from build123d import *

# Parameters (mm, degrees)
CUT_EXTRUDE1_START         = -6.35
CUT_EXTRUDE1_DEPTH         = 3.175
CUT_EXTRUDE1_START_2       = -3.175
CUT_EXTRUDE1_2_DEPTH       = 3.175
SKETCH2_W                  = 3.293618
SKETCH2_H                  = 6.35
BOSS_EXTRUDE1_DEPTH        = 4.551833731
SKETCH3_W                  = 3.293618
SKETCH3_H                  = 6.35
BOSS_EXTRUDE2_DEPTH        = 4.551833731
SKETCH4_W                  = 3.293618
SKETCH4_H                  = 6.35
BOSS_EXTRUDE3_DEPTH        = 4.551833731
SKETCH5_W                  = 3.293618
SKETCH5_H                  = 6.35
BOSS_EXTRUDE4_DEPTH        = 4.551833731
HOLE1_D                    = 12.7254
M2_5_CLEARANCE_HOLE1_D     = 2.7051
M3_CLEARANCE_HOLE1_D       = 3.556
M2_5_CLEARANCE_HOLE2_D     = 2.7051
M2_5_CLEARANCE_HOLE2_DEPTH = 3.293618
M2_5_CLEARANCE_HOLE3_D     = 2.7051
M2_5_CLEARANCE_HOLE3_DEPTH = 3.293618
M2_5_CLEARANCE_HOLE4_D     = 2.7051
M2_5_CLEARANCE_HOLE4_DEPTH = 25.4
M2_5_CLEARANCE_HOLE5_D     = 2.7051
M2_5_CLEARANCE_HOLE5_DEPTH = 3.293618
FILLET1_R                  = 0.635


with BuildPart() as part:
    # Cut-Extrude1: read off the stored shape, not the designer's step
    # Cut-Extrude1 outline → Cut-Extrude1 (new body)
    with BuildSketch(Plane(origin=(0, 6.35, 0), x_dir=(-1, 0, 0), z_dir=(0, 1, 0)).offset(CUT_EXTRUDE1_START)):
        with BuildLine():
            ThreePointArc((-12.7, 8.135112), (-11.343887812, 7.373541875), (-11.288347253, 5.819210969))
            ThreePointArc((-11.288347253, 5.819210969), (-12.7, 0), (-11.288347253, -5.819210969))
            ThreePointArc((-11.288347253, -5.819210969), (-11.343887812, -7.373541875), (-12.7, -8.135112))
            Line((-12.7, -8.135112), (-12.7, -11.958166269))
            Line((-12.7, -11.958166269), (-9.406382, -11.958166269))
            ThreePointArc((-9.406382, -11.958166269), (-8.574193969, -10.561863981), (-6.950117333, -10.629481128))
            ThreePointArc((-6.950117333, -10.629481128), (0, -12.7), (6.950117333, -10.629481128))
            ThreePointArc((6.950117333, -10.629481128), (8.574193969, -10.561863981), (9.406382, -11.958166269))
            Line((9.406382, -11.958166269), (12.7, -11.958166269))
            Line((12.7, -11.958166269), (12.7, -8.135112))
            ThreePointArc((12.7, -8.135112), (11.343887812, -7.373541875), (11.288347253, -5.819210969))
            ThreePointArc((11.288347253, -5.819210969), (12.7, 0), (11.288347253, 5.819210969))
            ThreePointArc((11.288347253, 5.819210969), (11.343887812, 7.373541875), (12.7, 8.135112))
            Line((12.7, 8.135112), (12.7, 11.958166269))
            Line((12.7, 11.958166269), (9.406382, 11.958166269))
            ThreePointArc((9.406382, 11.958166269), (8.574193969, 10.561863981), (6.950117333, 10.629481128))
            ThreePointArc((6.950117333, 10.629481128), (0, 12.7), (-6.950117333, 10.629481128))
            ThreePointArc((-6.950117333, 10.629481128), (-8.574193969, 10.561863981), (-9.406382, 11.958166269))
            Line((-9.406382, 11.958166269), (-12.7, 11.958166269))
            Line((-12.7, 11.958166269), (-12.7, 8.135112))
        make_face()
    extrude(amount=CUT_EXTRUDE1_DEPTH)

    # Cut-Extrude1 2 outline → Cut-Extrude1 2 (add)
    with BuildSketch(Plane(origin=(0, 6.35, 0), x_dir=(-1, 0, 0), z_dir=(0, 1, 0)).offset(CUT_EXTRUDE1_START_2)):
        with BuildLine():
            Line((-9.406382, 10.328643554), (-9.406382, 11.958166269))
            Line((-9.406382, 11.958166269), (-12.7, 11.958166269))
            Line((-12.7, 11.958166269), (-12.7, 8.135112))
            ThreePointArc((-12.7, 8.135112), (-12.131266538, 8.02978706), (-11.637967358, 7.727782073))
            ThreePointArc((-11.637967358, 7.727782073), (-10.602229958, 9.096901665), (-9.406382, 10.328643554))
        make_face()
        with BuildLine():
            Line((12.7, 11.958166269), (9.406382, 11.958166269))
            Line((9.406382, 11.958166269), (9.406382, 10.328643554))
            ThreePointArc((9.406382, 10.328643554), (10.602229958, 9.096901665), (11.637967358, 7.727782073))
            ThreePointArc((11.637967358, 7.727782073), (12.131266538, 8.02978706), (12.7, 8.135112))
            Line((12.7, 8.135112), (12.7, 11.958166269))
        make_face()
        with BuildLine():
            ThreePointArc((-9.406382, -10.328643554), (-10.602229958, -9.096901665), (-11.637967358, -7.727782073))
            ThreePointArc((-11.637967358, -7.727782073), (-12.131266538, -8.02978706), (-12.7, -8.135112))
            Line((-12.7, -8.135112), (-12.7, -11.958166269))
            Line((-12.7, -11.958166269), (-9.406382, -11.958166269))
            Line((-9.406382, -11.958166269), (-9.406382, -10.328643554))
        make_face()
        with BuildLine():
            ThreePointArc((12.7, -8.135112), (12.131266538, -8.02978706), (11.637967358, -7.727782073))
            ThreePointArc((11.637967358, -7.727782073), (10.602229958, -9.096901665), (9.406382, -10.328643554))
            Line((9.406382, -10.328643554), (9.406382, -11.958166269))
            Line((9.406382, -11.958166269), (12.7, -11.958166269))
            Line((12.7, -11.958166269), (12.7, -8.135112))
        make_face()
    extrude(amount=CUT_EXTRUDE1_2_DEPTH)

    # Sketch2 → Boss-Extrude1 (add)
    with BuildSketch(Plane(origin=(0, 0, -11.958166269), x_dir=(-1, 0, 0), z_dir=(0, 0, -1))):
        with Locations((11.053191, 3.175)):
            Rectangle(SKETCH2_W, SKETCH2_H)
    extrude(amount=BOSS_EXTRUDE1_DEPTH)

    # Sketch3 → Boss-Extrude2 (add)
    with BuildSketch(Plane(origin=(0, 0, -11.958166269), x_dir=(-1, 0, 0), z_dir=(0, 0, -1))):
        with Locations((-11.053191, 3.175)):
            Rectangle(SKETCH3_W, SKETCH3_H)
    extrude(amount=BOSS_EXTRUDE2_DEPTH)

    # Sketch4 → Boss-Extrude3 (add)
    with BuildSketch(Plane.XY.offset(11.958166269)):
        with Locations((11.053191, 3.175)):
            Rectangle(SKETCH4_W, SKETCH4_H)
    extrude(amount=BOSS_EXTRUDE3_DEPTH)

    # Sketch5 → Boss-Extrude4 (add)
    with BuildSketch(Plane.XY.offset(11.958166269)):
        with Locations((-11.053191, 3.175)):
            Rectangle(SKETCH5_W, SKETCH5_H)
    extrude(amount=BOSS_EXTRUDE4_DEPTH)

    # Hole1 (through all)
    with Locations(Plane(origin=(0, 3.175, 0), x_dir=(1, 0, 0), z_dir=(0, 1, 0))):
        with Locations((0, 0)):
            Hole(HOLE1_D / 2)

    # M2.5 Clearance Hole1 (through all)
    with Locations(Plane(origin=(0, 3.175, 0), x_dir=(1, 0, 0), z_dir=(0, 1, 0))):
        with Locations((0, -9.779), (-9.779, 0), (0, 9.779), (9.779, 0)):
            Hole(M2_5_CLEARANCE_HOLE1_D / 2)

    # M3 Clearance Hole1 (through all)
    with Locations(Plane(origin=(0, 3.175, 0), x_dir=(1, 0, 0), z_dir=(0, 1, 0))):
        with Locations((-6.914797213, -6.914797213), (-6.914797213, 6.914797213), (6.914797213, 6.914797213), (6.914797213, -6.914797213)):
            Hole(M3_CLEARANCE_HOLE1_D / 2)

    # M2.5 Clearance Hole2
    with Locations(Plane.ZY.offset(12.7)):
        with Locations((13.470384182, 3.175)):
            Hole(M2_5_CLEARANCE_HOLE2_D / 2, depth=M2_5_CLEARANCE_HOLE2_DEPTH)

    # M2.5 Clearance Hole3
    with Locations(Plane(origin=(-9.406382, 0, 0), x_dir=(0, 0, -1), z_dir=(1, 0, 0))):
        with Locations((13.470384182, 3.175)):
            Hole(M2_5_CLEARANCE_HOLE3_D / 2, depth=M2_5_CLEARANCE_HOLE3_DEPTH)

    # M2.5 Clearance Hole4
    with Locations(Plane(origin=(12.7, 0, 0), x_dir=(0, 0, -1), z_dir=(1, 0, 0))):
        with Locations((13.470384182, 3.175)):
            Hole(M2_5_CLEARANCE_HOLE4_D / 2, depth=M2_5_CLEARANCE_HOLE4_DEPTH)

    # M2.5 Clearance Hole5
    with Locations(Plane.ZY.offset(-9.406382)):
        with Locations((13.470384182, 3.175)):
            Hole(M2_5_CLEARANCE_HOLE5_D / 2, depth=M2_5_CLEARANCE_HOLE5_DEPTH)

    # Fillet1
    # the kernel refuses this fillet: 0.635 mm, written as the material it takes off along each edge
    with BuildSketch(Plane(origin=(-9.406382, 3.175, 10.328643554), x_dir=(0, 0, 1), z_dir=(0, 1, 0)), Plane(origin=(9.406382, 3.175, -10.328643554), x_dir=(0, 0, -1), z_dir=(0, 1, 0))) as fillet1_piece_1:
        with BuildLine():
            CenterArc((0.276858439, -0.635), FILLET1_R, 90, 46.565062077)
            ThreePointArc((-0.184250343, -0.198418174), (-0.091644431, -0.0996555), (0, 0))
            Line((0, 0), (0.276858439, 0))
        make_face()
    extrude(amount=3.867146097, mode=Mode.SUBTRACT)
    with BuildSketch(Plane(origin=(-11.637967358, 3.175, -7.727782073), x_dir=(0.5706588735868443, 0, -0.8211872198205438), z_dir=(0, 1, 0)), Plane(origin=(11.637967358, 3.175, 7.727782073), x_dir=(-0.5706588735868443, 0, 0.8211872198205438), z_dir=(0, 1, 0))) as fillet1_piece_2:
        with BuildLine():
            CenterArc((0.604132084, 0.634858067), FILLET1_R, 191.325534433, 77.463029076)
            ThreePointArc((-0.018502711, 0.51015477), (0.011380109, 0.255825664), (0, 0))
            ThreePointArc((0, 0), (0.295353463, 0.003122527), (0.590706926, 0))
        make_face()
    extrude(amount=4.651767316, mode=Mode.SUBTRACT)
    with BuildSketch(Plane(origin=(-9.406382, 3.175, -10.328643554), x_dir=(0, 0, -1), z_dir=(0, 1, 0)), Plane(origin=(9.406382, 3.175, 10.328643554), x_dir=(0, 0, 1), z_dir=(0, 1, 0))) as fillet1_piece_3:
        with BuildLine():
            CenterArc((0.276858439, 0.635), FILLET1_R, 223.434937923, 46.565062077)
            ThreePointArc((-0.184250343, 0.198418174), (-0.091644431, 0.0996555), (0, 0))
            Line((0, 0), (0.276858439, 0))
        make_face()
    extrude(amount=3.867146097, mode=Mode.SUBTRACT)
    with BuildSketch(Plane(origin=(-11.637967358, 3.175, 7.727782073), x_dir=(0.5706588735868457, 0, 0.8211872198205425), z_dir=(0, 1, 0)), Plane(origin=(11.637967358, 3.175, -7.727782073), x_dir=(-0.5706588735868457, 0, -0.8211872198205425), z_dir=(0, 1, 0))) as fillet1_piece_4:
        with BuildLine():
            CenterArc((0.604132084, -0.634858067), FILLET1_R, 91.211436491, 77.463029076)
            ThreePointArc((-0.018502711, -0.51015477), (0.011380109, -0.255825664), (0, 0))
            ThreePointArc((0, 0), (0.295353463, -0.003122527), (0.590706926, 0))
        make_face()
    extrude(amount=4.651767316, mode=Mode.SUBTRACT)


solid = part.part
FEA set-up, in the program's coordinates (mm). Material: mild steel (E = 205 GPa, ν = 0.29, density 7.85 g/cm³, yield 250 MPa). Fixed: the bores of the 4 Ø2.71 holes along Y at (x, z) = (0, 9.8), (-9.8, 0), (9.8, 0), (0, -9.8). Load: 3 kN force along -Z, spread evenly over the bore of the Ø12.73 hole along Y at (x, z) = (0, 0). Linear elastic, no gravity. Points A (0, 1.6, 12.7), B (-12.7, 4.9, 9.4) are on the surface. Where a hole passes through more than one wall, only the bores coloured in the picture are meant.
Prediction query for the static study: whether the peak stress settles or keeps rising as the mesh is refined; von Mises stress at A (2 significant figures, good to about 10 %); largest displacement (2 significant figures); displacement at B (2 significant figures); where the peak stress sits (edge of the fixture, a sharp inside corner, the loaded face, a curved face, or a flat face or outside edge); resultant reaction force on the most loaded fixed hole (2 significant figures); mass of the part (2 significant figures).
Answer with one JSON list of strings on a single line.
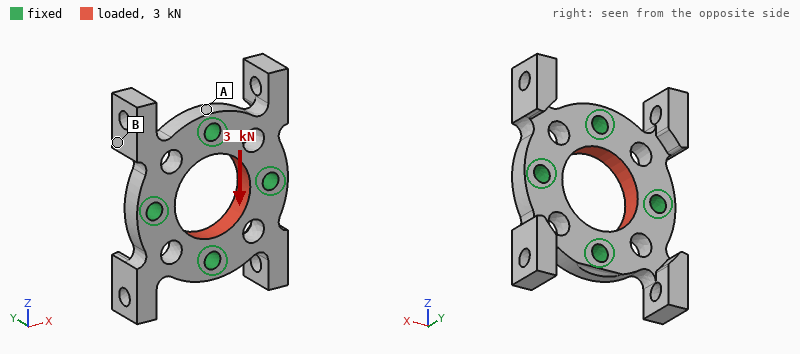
["keeps rising", "21 MPa", "1.7 µm", "0.61 µm", "edge of the fixture", "770 N", "13 g"]
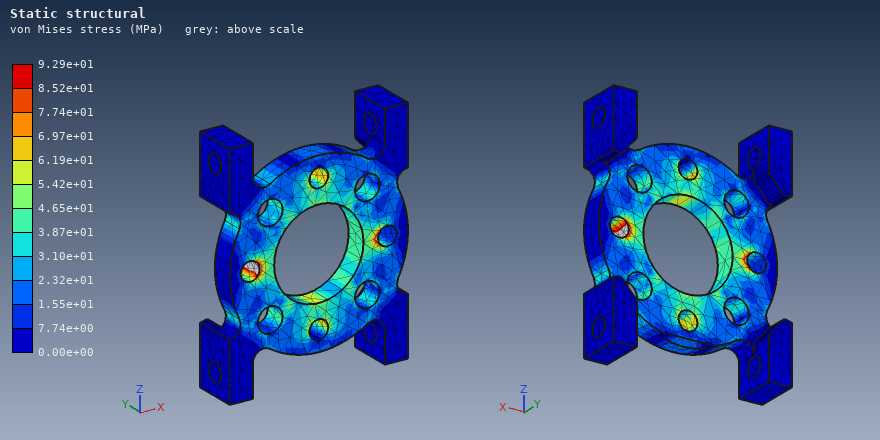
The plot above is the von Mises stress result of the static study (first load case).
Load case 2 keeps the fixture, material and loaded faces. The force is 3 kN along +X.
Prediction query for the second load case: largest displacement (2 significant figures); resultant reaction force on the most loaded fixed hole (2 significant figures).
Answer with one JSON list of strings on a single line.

["1.7 µm", "760 N"]
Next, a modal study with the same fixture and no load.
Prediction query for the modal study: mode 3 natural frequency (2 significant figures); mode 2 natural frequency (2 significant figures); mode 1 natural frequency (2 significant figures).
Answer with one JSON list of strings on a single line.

["12 kHz", "12 kHz", "12 kHz"]
